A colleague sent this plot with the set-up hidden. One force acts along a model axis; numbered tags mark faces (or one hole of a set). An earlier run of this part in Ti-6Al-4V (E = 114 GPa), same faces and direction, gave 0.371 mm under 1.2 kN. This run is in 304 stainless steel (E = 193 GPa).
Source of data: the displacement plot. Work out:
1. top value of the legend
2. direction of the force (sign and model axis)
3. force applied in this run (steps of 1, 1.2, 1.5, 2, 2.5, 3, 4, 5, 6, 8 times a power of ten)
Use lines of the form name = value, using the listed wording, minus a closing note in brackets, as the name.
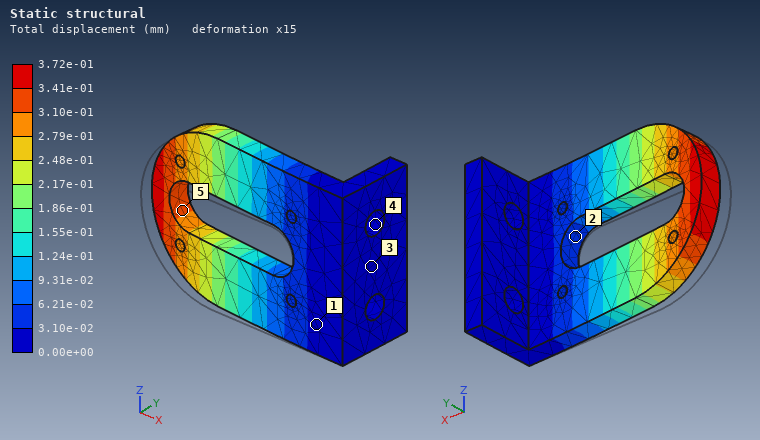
top value of the legend = 3.72e-01 mm
direction of the force = +Y
force applied in this run = 2 kN
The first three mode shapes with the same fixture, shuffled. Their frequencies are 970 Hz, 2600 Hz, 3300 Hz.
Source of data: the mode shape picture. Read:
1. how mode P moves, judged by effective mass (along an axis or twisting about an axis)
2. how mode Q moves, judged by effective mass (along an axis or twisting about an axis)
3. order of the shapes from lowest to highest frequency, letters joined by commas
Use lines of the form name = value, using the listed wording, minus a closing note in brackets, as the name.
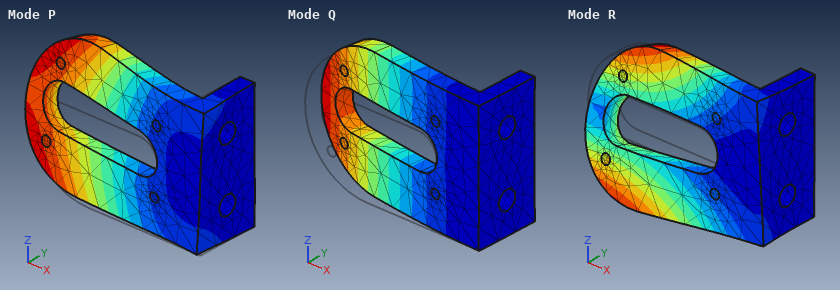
how mode P moves, judged by effective mass = along Z
how mode Q moves, judged by effective mass = along Y
order of the shapes from lowest to highest frequency, letters joined by commas = Q, R, P
